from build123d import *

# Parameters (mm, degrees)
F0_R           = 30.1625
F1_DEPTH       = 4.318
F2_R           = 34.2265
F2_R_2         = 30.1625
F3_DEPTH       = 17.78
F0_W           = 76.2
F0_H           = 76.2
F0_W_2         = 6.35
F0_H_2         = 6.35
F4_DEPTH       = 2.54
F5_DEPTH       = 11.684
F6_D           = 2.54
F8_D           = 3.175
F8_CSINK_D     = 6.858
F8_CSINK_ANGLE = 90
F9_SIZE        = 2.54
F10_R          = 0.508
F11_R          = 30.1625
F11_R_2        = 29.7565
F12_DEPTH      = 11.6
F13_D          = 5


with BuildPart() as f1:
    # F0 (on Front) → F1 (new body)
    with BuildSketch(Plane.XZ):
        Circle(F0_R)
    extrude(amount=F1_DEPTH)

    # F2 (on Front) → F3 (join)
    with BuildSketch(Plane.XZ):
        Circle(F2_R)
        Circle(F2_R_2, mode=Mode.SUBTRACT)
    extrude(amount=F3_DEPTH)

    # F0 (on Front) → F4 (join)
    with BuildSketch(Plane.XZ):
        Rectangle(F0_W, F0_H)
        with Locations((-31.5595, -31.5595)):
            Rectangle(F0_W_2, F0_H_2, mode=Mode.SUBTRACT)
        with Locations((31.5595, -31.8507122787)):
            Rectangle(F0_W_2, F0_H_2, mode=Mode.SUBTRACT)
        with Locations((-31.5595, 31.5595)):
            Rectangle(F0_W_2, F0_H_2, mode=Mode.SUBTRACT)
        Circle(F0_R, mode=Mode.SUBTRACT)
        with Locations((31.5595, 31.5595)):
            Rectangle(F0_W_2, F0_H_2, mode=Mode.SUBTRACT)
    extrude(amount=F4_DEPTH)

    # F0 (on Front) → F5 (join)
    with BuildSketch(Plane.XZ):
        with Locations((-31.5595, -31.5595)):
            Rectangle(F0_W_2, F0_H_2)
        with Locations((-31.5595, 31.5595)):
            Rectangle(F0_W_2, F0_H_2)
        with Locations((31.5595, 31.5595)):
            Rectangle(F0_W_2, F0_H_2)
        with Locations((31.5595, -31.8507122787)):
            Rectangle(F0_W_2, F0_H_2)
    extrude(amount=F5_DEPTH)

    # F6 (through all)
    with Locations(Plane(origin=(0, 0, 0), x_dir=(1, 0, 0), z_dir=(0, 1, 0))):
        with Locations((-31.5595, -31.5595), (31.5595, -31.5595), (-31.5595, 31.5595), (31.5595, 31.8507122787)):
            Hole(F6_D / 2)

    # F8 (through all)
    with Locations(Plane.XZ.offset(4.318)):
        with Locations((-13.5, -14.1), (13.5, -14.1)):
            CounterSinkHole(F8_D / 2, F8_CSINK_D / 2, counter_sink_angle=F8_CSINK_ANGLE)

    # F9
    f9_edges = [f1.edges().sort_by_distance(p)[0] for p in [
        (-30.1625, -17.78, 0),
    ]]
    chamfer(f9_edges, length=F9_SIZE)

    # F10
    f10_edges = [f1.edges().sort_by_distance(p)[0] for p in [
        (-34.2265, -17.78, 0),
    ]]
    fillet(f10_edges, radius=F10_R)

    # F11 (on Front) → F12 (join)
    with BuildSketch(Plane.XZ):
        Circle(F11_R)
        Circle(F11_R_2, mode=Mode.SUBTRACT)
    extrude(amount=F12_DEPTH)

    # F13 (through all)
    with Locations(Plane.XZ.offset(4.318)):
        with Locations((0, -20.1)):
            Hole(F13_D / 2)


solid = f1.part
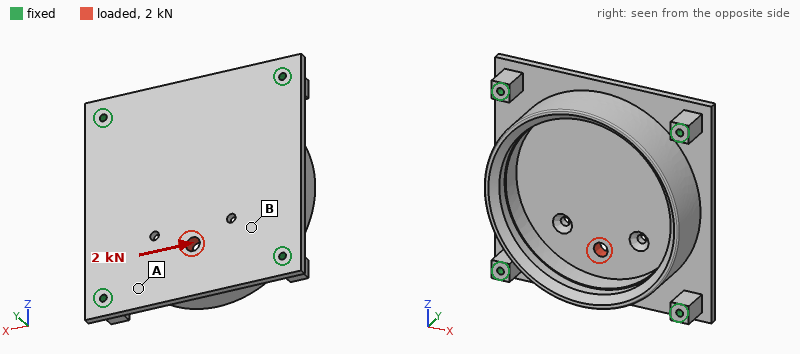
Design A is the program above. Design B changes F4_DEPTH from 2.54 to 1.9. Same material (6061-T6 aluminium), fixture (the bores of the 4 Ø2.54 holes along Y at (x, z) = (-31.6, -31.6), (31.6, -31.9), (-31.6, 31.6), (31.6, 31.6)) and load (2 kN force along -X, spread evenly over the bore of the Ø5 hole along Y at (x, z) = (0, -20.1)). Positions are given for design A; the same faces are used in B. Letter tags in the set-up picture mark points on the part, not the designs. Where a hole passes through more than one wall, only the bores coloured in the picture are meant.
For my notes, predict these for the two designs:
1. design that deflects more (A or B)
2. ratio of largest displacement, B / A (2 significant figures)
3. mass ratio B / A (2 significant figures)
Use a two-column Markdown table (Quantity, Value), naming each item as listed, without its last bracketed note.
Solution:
| Quantity | Value |
|---|---|
| design that deflects more | B |
| ratio of largest displacement, B / A | 1.2 |
| mass ratio B / A | 0.96 |
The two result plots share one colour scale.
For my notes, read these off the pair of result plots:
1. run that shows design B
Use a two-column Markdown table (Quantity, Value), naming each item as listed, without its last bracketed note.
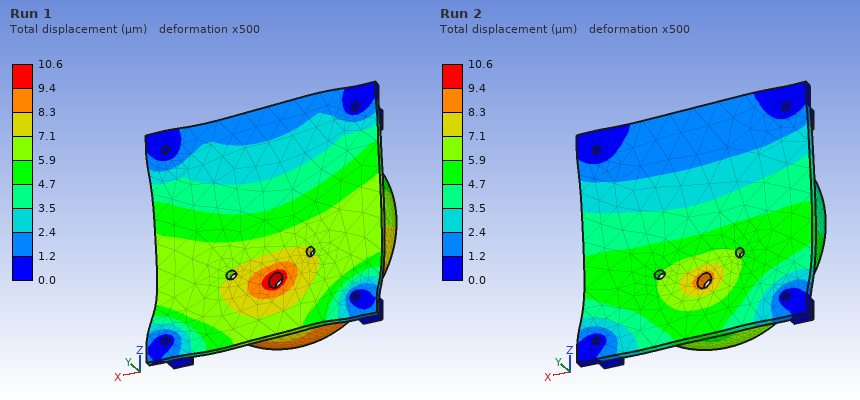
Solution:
| Quantity | Value |
|---|---|
| run that shows design B | Run 1 |
